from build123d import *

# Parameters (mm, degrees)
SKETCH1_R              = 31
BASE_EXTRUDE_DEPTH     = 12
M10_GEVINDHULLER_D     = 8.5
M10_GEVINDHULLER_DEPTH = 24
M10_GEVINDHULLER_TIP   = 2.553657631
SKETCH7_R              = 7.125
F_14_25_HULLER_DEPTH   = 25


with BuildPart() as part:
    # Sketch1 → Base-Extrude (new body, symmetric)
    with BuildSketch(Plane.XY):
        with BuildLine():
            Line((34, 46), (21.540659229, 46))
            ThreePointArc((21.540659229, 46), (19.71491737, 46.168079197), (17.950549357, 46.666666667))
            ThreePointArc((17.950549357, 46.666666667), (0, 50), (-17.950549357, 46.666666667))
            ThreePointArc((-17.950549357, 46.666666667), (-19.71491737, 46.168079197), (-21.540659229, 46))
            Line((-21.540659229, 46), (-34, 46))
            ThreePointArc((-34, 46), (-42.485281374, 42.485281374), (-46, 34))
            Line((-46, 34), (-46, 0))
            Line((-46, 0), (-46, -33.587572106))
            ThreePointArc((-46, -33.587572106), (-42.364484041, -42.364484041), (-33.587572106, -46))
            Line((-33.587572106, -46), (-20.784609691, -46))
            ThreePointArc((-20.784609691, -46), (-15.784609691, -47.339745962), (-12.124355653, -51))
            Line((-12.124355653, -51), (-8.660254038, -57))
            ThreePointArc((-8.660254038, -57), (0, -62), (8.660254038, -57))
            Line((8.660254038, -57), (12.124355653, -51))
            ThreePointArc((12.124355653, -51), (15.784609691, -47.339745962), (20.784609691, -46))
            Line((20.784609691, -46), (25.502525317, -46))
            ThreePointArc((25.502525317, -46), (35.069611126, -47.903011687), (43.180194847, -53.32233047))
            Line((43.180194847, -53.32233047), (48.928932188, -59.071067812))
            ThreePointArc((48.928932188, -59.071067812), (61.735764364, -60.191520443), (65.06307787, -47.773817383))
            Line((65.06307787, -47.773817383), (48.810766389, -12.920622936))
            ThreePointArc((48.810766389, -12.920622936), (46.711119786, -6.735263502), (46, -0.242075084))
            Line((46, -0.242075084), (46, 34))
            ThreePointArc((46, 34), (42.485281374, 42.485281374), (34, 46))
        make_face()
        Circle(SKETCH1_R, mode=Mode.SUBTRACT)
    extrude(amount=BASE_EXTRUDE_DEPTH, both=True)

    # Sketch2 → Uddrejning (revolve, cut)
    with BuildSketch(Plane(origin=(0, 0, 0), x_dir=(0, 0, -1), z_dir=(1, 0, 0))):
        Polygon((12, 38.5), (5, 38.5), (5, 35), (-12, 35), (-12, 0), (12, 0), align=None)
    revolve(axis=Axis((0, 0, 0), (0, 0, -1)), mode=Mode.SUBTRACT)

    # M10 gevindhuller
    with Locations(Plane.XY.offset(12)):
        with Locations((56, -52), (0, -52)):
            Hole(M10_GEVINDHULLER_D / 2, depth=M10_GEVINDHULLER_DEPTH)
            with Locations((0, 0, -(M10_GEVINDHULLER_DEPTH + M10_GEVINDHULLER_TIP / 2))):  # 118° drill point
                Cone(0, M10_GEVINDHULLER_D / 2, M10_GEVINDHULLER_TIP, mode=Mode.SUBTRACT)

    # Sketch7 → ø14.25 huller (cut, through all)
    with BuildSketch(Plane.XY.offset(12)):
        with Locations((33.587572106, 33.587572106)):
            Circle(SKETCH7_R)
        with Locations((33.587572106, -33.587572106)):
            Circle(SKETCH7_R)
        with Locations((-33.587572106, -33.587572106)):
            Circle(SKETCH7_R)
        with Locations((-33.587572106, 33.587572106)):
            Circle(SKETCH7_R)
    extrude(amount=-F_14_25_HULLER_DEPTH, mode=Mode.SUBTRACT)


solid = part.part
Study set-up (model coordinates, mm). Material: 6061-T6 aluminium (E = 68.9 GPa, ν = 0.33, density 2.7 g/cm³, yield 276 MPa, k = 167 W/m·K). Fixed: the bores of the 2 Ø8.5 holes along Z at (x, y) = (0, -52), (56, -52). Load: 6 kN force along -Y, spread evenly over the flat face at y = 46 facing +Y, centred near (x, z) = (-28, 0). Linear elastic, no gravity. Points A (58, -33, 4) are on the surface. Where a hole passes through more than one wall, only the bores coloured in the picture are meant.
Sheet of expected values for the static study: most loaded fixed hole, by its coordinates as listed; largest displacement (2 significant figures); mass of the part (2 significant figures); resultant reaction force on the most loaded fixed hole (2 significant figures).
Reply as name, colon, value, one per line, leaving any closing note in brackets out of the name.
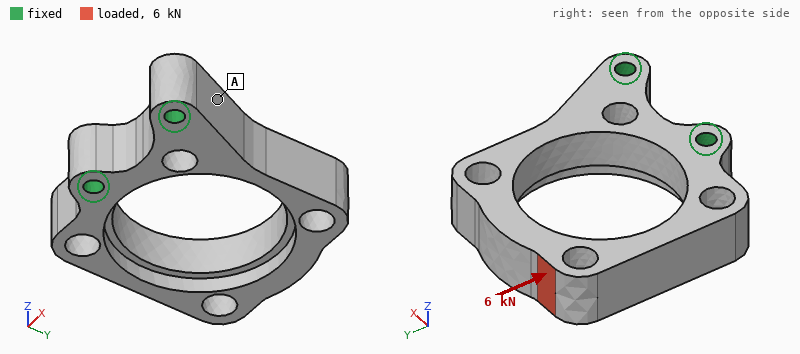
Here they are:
most loaded fixed hole, by its coordinates as listed: (0, -52)
largest displacement: 0.31 mm
mass of the part: 300 g
resultant reaction force on the most loaded fixed hole: 7.5 kN
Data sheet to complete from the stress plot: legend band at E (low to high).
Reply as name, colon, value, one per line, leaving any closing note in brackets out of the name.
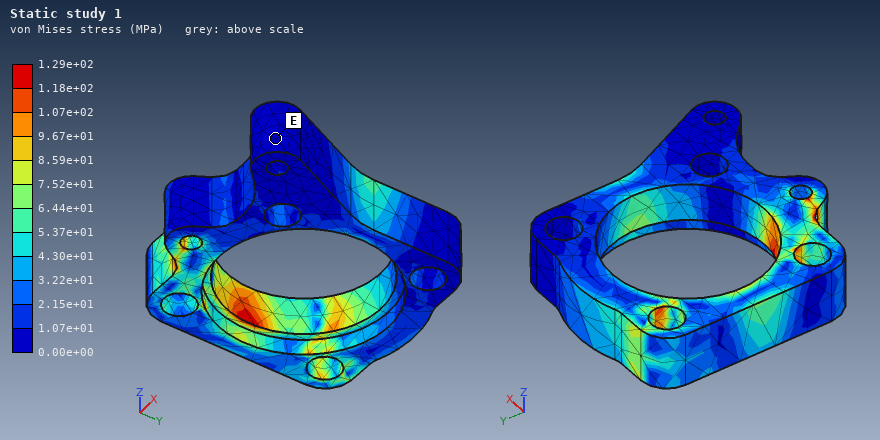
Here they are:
legend band at E: 0.00e+00 to 1.07e+01 MPa
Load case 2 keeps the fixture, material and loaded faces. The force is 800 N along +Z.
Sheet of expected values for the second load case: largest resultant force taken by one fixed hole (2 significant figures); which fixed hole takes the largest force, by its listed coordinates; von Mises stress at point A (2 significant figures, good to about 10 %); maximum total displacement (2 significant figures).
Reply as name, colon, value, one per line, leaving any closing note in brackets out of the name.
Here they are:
largest resultant force taken by one fixed hole: 770 N
which fixed hole takes the largest force, by its listed coordinates: (0, -52)
von Mises stress at point A: 4.9 MPa
maximum total displacement: 0.26 mm
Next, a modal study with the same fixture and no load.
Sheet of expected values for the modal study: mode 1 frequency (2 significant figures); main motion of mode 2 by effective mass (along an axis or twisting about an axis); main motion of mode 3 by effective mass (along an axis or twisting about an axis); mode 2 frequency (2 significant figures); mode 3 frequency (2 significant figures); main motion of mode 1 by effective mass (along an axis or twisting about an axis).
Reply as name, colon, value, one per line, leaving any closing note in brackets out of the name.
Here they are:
mode 1 frequency: 1200 Hz
main motion of mode 2 by effective mass: along X
main motion of mode 3 by effective mass: twisting about Y
mode 2 frequency: 1600 Hz
mode 3 frequency: 2700 Hz
main motion of mode 1 by effective mass: along Z
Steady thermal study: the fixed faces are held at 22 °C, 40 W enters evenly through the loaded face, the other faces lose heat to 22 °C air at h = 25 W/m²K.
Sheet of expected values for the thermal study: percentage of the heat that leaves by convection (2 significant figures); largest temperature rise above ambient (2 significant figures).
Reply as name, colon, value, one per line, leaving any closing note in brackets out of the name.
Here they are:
percentage of the heat that leaves by convection: 27 %
largest temperature rise above ambient: 44 K
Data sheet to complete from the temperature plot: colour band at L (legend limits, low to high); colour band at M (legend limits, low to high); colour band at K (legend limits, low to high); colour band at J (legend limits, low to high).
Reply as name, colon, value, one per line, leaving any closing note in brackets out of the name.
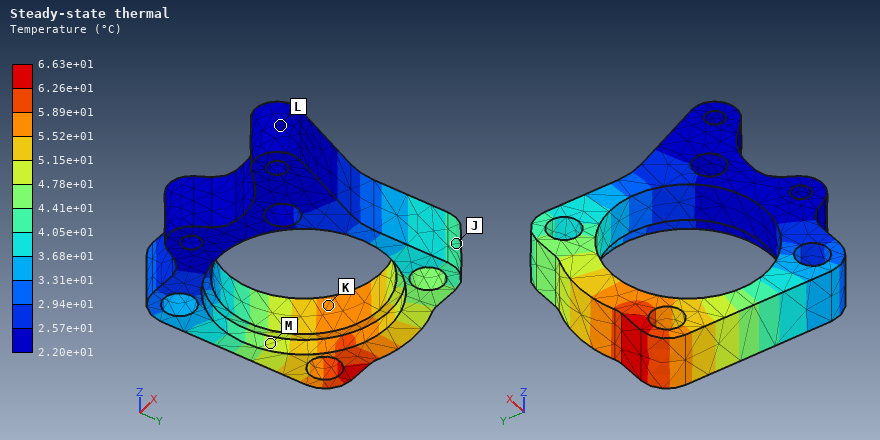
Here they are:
colour band at L: 2.20e+01 to 2.57e+01 °C
colour band at M: 4.78e+01 to 5.15e+01 °C
colour band at K: 5.52e+01 to 5.89e+01 °C
colour band at J: 4.05e+01 to 4.41e+01 °C
